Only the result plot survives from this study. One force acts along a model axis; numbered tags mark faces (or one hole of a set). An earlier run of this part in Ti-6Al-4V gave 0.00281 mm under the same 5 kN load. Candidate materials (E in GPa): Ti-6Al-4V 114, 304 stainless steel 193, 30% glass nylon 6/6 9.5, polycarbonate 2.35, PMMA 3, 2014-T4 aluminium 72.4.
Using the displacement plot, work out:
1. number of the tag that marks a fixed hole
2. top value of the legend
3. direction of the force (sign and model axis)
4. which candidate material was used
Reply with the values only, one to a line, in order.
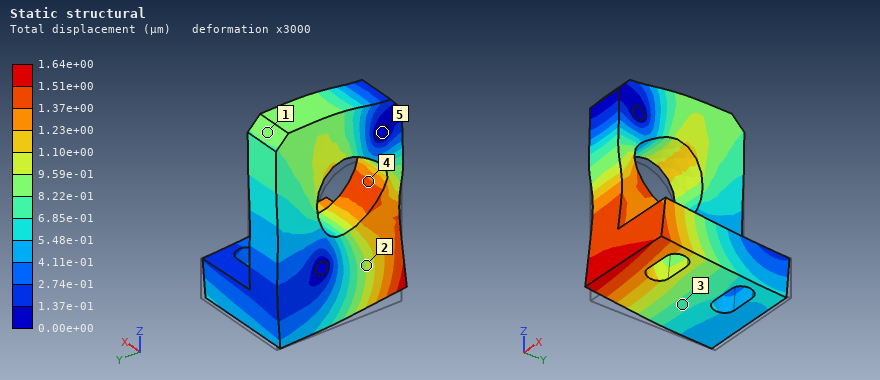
5
1.64e+00 µm
+Z
304 stainless steel
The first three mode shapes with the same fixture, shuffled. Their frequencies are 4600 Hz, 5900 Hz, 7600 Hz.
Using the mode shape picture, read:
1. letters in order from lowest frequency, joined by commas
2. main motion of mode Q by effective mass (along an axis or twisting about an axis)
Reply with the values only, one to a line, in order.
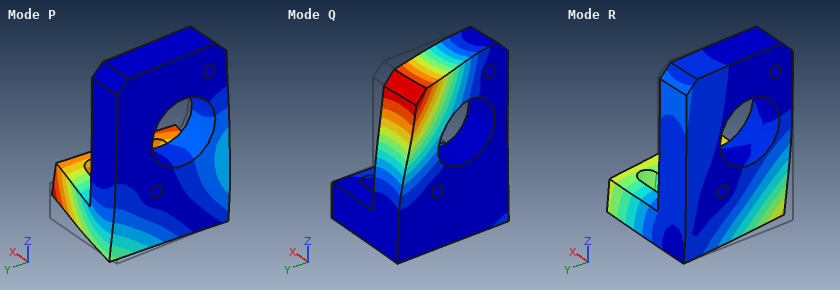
R, P, Q
along X
